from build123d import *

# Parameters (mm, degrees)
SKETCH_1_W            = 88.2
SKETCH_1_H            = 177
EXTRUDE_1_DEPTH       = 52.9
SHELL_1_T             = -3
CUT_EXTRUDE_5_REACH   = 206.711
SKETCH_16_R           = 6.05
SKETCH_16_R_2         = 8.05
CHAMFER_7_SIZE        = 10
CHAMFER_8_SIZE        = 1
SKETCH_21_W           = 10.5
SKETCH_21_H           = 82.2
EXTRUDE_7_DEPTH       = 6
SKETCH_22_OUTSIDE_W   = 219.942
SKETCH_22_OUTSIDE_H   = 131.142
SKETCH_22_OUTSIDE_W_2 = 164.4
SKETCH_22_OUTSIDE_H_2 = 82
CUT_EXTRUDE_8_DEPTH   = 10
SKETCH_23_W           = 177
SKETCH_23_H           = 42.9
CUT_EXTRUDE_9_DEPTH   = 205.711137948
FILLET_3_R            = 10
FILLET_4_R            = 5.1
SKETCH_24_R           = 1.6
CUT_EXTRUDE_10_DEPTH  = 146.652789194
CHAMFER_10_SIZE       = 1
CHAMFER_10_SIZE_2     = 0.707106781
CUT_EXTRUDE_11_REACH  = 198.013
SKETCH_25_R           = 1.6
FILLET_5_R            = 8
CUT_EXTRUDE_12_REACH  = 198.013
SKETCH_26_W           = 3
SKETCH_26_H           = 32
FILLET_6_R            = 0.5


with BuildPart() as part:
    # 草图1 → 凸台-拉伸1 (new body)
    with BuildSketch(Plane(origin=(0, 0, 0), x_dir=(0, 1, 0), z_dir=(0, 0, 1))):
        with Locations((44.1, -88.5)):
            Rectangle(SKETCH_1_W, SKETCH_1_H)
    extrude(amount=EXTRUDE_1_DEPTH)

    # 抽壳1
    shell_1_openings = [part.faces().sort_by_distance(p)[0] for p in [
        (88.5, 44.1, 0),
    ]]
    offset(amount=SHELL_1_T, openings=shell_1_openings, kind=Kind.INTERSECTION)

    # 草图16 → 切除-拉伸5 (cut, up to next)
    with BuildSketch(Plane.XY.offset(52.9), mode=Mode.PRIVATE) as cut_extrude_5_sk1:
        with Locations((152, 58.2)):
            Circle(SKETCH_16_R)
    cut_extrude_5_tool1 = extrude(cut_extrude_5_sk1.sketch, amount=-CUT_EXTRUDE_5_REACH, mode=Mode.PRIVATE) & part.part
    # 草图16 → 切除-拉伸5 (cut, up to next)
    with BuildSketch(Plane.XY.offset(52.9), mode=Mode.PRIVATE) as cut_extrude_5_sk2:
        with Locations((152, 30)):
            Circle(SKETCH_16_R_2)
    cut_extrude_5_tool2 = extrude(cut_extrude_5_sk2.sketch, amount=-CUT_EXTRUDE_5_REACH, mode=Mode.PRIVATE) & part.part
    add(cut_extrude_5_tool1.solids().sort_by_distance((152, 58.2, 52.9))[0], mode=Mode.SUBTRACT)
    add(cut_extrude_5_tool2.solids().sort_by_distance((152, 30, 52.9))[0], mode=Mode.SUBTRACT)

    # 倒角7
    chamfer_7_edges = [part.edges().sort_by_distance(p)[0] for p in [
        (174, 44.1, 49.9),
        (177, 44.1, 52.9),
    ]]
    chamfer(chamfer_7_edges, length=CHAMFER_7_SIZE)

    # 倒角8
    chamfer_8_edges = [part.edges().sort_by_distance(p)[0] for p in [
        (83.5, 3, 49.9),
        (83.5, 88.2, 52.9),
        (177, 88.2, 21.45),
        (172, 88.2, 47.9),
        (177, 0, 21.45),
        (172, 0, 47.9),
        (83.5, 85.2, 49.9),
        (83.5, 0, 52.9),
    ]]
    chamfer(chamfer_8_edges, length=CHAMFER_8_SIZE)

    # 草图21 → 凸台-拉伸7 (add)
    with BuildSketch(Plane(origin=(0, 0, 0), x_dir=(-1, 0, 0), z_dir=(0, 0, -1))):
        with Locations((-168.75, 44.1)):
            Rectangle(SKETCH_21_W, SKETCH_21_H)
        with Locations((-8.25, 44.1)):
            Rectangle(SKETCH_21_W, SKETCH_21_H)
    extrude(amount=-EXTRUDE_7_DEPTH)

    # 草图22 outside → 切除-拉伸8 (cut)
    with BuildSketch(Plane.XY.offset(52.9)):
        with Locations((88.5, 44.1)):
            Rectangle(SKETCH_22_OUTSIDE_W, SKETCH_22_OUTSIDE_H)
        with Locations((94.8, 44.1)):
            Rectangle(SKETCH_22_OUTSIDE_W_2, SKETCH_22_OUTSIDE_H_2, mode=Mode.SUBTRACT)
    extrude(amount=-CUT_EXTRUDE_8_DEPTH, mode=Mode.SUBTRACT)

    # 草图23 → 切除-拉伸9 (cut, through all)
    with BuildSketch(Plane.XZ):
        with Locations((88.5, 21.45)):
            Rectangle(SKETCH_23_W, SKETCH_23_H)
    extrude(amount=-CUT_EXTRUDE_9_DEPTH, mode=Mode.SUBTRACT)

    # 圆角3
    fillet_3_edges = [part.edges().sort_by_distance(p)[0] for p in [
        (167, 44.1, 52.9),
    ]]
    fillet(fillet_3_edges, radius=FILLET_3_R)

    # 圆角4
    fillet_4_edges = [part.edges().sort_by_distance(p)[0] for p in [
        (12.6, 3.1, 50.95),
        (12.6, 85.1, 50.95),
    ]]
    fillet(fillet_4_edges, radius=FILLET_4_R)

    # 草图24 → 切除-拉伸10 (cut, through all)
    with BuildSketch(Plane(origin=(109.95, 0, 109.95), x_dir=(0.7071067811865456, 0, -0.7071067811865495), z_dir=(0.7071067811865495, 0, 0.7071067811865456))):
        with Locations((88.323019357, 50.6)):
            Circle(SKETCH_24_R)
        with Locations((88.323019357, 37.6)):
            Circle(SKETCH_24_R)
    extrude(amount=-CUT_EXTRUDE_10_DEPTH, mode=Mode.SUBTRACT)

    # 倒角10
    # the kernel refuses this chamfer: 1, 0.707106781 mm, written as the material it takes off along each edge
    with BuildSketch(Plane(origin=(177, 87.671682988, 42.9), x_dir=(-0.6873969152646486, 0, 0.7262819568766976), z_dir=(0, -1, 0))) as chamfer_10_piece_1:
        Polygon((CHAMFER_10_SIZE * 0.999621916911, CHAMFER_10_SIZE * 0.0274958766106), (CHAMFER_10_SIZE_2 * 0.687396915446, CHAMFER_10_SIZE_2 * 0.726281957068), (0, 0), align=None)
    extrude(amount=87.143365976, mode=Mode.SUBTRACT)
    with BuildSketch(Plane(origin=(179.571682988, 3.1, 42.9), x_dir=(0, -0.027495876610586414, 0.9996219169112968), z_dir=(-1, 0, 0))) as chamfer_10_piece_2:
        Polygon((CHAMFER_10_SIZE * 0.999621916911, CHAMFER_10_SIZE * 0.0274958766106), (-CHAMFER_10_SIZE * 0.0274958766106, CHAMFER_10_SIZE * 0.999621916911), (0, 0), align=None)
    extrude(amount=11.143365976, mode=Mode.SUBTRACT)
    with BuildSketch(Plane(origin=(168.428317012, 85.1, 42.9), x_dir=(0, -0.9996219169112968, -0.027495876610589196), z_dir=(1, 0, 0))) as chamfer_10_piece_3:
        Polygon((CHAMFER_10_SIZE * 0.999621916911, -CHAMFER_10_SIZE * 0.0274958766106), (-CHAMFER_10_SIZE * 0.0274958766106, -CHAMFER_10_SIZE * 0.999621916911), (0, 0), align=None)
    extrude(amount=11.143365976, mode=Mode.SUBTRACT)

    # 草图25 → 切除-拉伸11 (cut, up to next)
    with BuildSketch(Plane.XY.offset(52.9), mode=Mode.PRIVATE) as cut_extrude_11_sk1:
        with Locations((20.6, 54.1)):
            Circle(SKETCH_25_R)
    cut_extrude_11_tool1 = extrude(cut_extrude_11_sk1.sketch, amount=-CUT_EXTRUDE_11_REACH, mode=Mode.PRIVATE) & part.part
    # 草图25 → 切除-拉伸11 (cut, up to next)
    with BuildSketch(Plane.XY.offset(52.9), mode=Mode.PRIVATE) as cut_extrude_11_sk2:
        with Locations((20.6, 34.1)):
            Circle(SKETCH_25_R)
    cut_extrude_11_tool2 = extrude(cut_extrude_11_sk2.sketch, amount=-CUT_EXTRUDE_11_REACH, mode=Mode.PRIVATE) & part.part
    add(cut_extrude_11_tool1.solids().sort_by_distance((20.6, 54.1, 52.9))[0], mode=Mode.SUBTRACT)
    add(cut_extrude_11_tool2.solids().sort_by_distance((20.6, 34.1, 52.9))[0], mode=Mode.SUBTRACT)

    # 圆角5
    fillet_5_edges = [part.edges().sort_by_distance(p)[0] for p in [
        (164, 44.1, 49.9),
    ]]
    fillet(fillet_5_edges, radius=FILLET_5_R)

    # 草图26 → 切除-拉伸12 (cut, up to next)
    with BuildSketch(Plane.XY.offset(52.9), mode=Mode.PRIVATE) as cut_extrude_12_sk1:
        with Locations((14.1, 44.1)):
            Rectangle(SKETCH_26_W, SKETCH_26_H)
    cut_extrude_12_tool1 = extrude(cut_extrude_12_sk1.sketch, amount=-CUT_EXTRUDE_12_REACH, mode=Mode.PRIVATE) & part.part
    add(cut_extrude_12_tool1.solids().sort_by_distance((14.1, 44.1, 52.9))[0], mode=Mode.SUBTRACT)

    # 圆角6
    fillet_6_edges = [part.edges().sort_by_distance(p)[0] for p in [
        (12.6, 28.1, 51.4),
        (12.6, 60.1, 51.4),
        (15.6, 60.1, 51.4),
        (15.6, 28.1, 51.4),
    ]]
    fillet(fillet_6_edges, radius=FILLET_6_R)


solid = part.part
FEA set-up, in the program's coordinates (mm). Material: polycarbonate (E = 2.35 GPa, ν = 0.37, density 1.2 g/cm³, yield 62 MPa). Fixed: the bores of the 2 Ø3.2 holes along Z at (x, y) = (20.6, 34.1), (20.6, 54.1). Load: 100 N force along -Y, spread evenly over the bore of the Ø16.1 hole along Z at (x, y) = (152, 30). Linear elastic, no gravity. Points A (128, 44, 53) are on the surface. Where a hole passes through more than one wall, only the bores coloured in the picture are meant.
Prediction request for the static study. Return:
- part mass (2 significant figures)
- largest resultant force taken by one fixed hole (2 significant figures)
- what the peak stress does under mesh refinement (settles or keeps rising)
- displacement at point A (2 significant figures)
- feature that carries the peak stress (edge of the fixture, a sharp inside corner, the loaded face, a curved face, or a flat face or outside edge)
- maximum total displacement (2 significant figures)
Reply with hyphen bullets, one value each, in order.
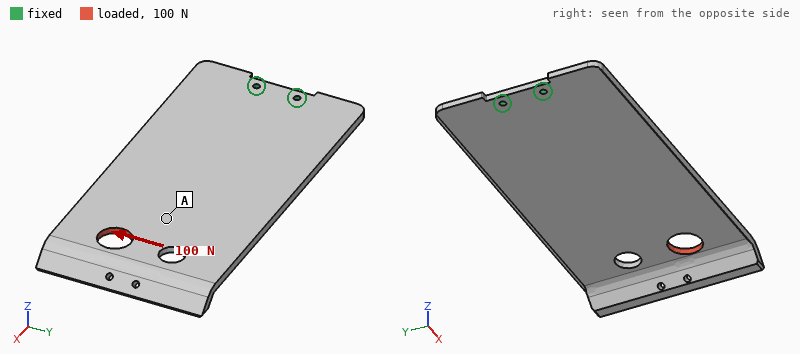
- 49 g
- 590 N
- keeps rising
- 1.3 mm
- edge of the fixture
- 1.9 mm
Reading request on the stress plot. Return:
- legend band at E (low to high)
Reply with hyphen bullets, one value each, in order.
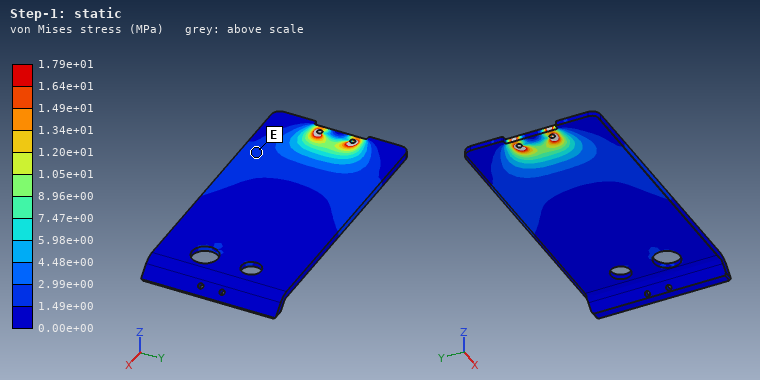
- 1.49e+00 to 2.99e+00 MPa
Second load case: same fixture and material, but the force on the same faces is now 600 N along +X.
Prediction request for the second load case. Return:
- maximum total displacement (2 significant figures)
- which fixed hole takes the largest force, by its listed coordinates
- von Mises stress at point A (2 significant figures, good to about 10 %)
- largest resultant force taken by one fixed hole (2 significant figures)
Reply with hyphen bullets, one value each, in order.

- 1.4 mm
- (20.6, 34.1)
- 3.4 MPa
- 680 N
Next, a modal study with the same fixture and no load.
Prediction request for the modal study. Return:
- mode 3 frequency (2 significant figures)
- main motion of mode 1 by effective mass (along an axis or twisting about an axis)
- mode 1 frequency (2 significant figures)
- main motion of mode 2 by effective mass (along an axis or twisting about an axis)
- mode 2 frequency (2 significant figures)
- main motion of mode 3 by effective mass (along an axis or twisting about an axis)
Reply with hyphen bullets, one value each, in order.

- 160 Hz
- along Z
- 26 Hz
- twisting about X
- 97 Hz
- along Z
